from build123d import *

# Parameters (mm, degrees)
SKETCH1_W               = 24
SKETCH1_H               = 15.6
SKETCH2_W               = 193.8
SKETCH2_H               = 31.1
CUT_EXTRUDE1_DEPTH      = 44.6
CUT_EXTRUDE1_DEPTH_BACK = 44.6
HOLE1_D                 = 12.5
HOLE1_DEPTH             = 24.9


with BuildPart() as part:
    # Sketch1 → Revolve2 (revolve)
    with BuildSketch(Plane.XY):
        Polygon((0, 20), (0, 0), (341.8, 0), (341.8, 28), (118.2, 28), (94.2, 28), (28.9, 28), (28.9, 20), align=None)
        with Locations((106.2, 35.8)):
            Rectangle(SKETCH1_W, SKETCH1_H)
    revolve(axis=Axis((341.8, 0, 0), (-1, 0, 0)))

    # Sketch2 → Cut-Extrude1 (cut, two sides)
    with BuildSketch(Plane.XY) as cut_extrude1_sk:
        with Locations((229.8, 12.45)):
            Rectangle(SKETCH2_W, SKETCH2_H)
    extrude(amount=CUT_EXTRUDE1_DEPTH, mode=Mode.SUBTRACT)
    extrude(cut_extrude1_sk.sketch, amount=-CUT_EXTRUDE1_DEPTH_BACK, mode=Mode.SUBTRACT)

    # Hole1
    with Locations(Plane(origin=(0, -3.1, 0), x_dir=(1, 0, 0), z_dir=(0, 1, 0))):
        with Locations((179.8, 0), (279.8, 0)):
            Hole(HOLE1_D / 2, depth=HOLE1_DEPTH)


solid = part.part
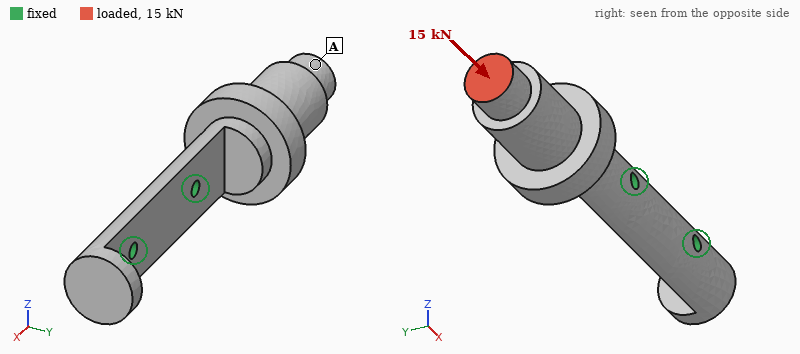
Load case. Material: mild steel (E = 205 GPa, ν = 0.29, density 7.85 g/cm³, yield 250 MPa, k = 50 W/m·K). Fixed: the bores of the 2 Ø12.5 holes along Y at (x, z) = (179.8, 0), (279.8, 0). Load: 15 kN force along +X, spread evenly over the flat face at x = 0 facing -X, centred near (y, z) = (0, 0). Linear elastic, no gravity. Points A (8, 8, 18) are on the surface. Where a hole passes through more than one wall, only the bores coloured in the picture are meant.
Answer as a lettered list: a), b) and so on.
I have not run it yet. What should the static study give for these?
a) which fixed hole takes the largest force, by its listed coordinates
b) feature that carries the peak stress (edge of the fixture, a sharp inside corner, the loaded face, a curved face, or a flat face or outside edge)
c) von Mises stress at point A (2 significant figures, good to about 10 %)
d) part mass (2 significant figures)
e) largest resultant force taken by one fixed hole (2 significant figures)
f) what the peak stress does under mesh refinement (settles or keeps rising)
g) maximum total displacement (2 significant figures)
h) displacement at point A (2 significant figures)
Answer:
a) (179.8, 0)
b) edge of the fixture
c) 12 MPa
d) 4.8 kg
e) 13 kN
f) keeps rising
g) 0.19 mm
h) 0.18 mm
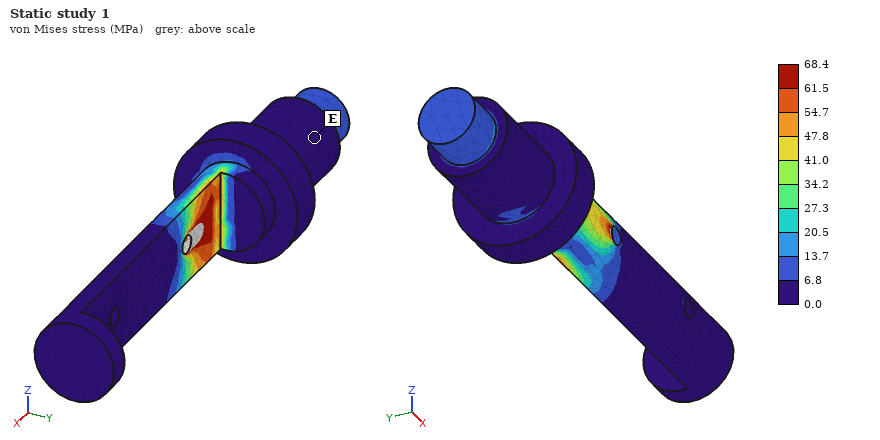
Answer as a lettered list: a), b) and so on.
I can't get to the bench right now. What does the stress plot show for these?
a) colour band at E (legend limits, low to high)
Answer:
a) 0.0 to 6.8 MPa
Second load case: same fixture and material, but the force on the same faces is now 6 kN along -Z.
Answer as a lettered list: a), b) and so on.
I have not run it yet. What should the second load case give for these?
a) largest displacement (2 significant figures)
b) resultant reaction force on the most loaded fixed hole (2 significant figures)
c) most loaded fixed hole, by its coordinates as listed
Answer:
a) 0.34 mm
b) 12 kN
c) (179.8, 0)
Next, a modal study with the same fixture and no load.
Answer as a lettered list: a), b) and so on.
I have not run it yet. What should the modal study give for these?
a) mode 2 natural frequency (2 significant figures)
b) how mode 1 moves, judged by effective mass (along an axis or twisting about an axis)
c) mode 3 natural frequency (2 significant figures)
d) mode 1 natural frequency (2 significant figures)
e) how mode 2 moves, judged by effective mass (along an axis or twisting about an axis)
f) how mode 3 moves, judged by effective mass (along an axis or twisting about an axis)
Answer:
a) 710 Hz
b) along Y
c) 1700 Hz
d) 450 Hz
e) along Z
f) twisting about X
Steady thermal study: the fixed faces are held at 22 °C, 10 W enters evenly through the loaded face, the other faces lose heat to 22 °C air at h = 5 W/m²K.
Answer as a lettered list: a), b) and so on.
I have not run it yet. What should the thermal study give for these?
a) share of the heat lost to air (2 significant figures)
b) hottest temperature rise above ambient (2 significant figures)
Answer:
a) 21 %
b) 20 K
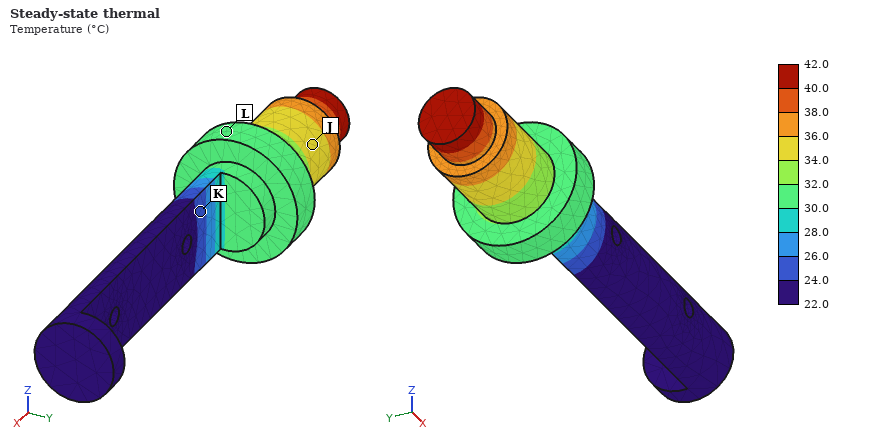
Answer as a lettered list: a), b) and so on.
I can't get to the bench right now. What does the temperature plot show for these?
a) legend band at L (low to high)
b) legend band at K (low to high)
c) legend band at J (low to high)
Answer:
a) 30.0 to 32.0 °C
b) 24.0 to 26.0 °C
c) 34.0 to 36.0 °C
